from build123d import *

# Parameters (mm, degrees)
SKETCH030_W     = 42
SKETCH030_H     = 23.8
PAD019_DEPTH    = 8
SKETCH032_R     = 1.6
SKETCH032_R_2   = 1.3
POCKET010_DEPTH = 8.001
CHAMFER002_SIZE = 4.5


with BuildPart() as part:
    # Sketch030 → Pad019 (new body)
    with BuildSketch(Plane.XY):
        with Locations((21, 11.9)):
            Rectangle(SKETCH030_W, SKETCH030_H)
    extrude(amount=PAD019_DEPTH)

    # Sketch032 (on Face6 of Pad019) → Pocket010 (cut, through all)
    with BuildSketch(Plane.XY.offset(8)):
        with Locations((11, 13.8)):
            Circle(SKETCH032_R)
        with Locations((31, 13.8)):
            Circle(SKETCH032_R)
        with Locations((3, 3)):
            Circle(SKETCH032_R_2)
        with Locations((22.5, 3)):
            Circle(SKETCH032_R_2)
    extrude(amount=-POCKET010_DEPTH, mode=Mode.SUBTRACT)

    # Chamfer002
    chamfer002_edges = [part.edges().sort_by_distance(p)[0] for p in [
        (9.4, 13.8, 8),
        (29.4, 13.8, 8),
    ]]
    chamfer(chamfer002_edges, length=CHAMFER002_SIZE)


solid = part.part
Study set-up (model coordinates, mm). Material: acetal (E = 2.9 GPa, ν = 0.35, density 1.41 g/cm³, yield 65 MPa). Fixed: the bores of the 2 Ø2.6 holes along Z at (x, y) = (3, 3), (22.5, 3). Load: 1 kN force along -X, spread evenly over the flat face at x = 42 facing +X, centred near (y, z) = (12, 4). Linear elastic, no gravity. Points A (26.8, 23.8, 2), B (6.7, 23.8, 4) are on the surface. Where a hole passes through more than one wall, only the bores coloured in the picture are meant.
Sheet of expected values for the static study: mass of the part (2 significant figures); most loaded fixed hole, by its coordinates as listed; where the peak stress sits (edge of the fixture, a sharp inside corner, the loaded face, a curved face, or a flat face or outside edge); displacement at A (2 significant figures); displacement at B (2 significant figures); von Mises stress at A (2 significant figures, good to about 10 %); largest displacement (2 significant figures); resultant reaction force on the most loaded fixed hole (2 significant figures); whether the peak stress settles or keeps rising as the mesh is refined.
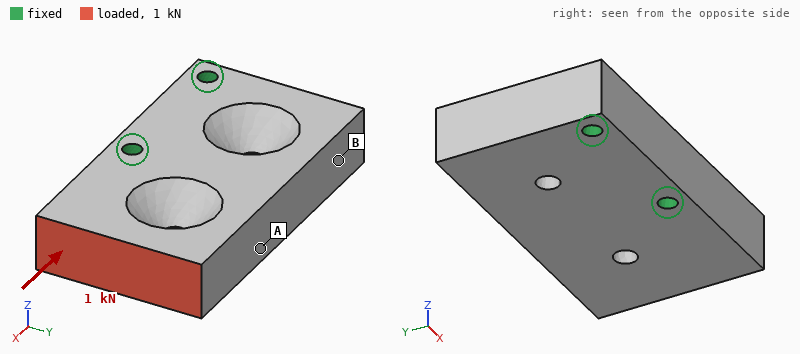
10 g
(22.5, 3)
edge of the fixture
0.13 mm
0.089 mm
6.9 MPa
0.21 mm
790 N
keeps rising
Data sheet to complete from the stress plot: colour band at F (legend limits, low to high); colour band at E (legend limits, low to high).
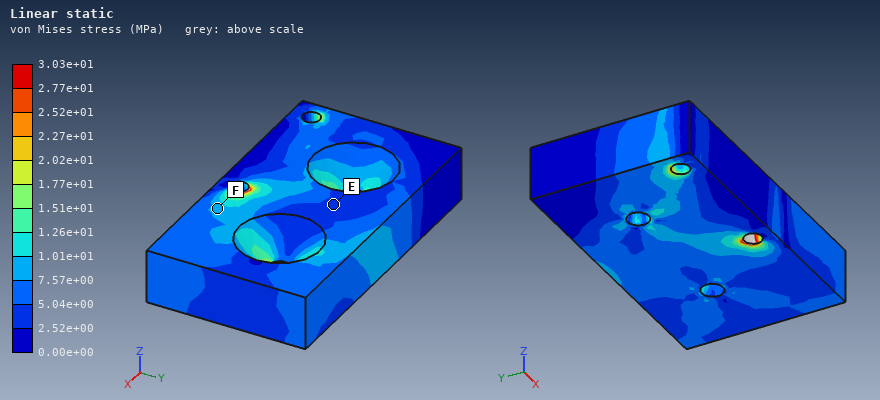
7.57e+00 to 1.01e+01 MPa
2.52e+00 to 5.04e+00 MPa
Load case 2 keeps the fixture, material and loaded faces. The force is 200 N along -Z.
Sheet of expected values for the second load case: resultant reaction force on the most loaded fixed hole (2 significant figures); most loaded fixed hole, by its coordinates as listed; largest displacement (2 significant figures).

280 N
(22.5, 3)
0.51 mm
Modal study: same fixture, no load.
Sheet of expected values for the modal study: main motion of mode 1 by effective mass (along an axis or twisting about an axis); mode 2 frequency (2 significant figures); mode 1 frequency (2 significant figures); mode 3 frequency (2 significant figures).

along Z
3500 Hz
2400 Hz
4100 Hz
